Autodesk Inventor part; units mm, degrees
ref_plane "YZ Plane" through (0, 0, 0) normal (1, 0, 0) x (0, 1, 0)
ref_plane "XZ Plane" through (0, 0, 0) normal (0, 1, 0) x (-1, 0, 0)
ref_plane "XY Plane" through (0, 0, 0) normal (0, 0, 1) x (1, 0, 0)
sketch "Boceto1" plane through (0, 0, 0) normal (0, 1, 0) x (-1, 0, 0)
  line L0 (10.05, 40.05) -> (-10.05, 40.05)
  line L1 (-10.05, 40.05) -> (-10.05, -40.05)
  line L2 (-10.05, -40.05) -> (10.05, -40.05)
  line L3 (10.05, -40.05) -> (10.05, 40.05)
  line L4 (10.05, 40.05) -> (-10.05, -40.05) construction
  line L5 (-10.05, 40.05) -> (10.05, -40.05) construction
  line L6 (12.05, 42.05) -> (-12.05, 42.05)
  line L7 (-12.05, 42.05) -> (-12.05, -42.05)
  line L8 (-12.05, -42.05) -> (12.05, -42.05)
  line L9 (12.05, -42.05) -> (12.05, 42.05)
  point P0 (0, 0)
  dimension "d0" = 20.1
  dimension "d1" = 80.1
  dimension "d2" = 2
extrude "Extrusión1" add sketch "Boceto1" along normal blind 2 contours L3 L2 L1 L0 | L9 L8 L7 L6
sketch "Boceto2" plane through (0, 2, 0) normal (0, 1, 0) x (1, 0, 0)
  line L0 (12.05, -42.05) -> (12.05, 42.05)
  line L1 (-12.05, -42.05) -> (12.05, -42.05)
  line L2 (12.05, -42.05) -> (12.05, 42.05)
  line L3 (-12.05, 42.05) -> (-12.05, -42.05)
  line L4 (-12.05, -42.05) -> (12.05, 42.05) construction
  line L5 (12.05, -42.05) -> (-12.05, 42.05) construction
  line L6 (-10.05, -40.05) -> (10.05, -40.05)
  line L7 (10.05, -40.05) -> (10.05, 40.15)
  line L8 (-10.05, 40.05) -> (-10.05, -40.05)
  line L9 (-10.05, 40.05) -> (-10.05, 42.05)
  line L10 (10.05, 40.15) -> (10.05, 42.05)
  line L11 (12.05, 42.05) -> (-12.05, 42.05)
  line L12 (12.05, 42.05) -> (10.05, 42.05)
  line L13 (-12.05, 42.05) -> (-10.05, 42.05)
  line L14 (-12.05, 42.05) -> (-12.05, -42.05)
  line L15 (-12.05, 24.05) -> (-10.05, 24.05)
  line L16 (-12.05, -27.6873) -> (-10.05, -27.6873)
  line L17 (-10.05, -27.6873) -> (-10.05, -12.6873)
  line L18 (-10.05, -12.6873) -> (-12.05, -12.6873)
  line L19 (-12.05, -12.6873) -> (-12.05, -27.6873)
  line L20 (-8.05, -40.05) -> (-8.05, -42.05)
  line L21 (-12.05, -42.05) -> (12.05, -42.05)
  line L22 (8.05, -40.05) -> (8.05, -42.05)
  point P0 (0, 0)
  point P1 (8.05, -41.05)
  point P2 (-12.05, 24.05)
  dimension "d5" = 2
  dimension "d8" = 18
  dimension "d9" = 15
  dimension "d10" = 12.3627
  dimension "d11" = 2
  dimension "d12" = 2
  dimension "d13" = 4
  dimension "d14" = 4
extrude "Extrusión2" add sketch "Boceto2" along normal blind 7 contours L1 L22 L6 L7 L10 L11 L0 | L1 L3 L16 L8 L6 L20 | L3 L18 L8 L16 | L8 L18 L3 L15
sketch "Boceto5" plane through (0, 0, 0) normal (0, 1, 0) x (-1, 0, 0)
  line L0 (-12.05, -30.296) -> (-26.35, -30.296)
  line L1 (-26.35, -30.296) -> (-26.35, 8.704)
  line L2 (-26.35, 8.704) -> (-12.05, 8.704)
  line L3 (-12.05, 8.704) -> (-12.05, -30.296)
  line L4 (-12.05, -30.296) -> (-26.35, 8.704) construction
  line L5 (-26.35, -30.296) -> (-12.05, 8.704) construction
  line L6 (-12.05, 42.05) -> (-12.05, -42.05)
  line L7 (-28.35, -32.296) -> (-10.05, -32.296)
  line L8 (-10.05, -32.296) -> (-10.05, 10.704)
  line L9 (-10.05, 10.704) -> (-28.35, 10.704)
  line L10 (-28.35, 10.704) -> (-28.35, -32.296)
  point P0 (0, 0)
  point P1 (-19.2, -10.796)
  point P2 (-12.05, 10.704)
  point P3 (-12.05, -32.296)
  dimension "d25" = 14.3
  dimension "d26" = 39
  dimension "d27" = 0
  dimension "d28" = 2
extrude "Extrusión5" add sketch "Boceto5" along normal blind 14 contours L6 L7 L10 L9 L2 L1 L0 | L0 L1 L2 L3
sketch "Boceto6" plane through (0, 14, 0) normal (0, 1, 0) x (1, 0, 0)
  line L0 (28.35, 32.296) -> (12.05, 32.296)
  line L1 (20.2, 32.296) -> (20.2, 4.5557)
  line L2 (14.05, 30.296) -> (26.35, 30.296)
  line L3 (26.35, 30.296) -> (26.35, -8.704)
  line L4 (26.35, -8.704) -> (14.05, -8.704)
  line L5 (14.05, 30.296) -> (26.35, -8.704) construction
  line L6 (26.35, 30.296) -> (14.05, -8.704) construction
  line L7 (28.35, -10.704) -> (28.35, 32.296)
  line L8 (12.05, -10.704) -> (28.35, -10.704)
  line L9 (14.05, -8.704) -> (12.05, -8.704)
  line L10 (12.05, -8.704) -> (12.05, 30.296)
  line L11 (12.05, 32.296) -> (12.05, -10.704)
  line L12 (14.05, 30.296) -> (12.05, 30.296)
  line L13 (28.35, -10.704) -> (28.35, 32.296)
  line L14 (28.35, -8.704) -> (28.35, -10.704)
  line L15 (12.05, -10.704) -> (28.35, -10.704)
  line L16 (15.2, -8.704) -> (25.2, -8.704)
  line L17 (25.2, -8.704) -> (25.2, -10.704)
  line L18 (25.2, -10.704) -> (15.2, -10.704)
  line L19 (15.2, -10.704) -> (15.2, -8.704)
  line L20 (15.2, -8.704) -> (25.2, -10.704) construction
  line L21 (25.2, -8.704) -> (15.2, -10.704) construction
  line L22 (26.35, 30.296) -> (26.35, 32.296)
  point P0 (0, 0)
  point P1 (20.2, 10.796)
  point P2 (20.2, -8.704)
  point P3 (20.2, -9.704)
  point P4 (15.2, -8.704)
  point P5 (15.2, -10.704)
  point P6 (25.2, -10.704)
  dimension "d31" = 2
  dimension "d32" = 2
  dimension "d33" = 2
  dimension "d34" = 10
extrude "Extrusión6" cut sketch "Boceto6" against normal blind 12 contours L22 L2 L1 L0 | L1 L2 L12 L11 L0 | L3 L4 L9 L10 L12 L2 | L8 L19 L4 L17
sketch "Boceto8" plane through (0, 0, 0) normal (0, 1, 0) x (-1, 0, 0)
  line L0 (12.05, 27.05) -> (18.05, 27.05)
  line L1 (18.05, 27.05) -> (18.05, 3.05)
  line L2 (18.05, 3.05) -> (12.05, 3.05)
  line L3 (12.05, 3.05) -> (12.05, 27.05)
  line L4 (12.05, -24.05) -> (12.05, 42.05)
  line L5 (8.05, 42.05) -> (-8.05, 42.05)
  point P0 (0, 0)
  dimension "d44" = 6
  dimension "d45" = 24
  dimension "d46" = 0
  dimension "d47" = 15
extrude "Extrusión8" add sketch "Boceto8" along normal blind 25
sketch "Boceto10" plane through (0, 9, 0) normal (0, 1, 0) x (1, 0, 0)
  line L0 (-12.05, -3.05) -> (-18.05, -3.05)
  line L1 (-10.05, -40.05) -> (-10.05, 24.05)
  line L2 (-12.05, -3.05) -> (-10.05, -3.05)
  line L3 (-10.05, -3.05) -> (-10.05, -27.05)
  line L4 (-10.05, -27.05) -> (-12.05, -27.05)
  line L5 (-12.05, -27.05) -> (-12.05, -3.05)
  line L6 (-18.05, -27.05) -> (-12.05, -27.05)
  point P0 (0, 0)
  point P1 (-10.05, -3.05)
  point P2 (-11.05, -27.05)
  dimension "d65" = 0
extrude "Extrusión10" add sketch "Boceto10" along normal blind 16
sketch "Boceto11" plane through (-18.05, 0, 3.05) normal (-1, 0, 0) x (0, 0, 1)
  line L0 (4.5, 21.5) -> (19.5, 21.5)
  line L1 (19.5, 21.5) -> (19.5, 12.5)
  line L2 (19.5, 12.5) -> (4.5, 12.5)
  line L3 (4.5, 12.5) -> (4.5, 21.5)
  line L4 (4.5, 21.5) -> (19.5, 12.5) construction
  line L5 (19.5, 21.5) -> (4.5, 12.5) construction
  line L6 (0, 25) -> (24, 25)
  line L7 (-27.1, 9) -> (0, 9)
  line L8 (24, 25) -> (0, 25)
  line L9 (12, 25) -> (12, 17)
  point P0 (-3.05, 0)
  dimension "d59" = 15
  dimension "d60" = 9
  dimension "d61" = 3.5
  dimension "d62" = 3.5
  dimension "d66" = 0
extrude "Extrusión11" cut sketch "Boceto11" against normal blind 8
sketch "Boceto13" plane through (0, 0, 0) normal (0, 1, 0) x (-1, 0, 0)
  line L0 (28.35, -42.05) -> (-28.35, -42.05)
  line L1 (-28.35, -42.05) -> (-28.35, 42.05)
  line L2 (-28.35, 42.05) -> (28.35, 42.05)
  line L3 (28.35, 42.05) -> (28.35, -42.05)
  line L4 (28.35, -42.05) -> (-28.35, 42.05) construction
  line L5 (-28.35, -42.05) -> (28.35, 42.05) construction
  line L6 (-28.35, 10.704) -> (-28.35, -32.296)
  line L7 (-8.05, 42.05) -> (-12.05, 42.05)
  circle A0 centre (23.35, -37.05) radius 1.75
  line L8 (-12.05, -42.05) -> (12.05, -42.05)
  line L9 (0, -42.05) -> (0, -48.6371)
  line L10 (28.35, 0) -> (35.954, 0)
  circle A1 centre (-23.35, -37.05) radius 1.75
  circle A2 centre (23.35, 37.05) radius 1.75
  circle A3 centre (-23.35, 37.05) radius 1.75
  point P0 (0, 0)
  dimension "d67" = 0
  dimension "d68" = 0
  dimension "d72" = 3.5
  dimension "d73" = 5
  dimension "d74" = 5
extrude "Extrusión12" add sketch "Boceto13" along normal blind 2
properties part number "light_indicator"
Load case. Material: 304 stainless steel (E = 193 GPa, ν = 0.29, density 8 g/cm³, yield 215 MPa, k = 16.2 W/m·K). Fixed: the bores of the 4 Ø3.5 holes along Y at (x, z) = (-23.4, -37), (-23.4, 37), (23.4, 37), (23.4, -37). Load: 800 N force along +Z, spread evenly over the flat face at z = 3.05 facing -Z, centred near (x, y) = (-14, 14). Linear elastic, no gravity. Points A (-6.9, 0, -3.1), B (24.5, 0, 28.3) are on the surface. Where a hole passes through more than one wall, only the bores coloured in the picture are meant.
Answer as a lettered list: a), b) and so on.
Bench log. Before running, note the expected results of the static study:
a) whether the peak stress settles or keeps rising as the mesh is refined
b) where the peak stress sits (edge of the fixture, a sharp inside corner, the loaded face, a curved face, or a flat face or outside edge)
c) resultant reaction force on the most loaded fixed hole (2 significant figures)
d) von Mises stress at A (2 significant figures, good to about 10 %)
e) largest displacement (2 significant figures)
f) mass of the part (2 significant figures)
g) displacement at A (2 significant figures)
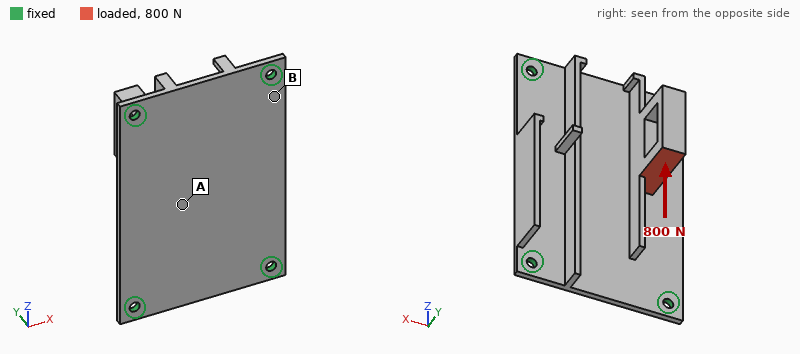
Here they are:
a) keeps rising
b) edge of the fixture
c) 310 N
d) 20 MPa
e) 48 µm
f) 130 g
g) 24 µm
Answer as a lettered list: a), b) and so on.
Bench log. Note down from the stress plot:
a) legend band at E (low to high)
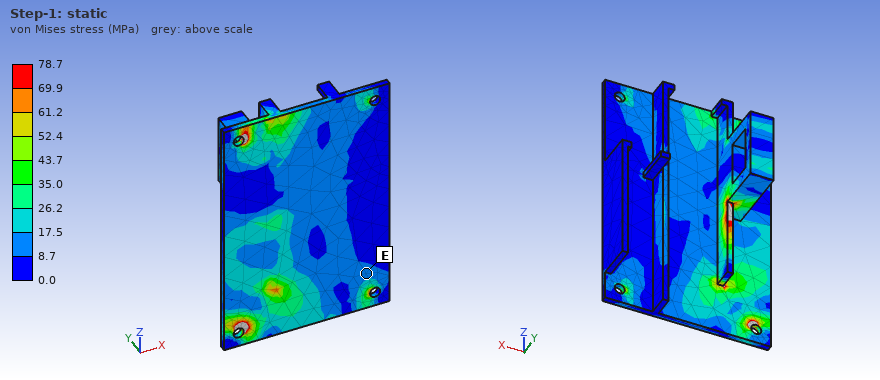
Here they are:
a) 8.7 to 17.5 MPa
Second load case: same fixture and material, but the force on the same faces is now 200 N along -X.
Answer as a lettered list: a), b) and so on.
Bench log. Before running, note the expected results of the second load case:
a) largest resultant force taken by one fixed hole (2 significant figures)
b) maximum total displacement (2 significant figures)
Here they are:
a) 100 N
b) 49 µm
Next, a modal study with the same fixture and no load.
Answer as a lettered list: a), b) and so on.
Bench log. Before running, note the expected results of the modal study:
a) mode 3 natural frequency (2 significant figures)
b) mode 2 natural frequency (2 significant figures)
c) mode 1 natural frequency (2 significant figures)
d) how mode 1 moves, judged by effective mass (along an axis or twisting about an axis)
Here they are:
a) 2900 Hz
b) 2400 Hz
c) 2100 Hz
d) along Y
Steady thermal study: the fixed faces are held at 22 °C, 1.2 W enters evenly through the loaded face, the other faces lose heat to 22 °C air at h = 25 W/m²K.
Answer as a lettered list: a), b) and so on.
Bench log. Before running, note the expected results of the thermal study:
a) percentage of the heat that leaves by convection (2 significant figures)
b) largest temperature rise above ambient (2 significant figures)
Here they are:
a) 75 %
b) 15 K
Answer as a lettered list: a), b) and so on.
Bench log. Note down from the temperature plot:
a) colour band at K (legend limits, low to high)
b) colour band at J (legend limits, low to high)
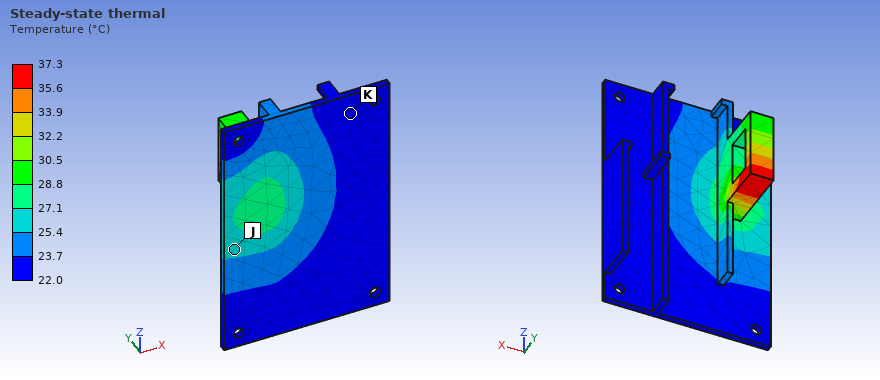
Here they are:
a) 22.0 to 23.7 °C
b) 25.4 to 27.1 °C
